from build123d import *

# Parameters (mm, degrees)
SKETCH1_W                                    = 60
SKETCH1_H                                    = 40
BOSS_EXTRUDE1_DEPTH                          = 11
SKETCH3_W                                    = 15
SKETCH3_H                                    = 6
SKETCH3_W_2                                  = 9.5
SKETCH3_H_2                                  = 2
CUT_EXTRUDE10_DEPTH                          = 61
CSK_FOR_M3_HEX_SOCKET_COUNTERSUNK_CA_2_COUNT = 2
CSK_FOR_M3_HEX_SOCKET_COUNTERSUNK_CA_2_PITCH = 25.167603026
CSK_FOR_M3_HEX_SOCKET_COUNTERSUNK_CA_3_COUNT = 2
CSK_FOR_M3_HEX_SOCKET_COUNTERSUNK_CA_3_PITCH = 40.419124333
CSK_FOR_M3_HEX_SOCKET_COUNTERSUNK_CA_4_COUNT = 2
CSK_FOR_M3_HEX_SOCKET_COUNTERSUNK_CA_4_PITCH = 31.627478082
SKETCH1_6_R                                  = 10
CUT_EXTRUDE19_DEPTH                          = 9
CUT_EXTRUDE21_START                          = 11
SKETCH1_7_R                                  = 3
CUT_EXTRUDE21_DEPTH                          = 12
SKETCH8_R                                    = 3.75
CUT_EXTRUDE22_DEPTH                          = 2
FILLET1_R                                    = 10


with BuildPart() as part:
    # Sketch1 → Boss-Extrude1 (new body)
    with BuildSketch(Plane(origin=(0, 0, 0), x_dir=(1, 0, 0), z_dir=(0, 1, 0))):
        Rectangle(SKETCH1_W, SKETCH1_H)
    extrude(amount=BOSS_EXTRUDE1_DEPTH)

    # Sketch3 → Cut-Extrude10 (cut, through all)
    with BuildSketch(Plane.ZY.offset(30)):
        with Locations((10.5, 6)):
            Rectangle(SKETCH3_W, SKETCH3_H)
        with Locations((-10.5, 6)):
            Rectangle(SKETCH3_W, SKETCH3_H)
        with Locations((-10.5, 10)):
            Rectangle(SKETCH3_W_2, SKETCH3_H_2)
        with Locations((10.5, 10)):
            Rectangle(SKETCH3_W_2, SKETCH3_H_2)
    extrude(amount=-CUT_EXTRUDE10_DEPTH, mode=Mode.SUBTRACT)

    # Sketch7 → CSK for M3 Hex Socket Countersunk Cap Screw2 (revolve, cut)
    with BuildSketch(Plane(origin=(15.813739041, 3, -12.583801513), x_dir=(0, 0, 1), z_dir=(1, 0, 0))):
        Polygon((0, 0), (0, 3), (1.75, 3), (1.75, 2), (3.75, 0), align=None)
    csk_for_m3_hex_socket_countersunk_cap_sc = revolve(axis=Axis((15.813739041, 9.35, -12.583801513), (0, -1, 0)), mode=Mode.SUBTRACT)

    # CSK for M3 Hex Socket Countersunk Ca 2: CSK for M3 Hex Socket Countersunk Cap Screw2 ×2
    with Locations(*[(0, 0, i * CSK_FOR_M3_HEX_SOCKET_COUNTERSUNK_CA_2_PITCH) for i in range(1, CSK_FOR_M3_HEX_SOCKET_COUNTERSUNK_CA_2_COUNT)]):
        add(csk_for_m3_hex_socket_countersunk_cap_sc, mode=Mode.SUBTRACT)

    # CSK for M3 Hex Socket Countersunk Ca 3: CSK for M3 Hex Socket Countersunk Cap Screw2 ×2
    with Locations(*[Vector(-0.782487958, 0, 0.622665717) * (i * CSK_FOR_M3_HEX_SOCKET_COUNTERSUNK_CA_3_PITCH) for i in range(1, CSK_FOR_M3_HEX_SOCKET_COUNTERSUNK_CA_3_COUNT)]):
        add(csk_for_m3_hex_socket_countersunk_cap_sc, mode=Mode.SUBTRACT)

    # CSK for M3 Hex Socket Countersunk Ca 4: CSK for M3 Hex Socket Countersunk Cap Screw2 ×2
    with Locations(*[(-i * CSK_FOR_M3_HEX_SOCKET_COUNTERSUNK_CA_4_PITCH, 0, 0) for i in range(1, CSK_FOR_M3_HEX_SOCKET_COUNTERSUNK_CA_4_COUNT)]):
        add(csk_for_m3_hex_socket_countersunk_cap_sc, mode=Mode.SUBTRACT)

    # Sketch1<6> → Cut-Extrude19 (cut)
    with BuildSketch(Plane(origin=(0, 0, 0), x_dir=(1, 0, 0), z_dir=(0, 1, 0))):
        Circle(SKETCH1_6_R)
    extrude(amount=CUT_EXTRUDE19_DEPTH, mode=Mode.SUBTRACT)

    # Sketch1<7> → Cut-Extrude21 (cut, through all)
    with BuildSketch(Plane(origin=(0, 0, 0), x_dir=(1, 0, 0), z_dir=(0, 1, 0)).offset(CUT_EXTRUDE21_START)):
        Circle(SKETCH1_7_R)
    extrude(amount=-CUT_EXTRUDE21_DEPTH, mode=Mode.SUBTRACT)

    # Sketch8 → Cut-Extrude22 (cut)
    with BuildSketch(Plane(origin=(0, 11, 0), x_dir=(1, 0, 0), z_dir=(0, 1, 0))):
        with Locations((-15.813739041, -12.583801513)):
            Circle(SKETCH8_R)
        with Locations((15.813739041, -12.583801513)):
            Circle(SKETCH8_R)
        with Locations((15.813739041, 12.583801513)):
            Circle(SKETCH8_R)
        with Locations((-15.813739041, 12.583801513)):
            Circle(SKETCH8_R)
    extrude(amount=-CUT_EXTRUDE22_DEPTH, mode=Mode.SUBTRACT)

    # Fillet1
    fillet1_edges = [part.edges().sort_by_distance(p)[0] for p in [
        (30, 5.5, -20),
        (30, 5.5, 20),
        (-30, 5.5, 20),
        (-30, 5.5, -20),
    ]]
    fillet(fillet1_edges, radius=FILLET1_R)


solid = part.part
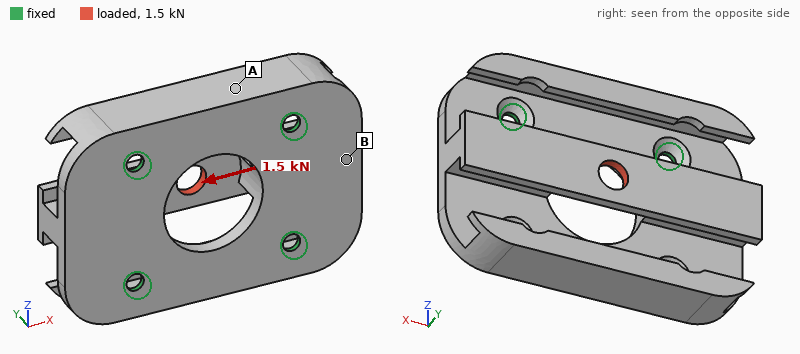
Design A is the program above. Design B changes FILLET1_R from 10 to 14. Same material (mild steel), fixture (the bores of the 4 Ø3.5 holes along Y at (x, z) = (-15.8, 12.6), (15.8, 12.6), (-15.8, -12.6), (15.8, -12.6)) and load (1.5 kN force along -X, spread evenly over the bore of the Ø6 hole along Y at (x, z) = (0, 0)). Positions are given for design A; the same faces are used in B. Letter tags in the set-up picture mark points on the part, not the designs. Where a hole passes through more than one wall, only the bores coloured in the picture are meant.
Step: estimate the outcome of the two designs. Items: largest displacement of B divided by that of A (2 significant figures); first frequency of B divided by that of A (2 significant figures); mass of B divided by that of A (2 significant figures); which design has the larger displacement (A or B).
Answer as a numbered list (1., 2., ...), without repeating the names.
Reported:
1. 1.1
2. 0.96
3. 0.95
4. B
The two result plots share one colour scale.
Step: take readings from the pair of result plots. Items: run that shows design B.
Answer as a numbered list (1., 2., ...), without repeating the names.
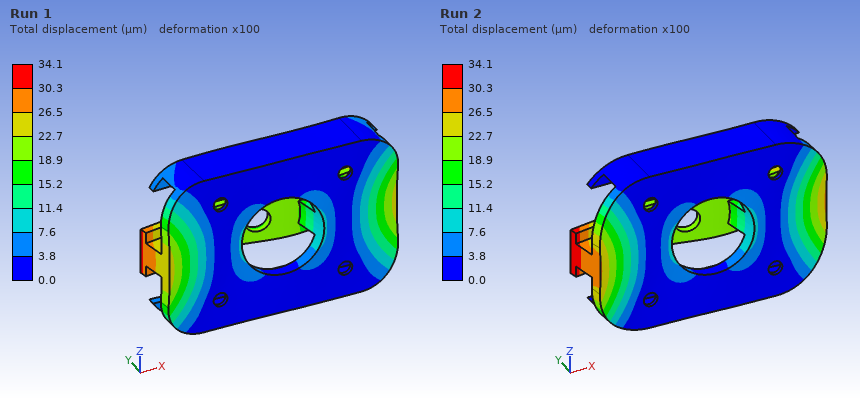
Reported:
1. Run 2
